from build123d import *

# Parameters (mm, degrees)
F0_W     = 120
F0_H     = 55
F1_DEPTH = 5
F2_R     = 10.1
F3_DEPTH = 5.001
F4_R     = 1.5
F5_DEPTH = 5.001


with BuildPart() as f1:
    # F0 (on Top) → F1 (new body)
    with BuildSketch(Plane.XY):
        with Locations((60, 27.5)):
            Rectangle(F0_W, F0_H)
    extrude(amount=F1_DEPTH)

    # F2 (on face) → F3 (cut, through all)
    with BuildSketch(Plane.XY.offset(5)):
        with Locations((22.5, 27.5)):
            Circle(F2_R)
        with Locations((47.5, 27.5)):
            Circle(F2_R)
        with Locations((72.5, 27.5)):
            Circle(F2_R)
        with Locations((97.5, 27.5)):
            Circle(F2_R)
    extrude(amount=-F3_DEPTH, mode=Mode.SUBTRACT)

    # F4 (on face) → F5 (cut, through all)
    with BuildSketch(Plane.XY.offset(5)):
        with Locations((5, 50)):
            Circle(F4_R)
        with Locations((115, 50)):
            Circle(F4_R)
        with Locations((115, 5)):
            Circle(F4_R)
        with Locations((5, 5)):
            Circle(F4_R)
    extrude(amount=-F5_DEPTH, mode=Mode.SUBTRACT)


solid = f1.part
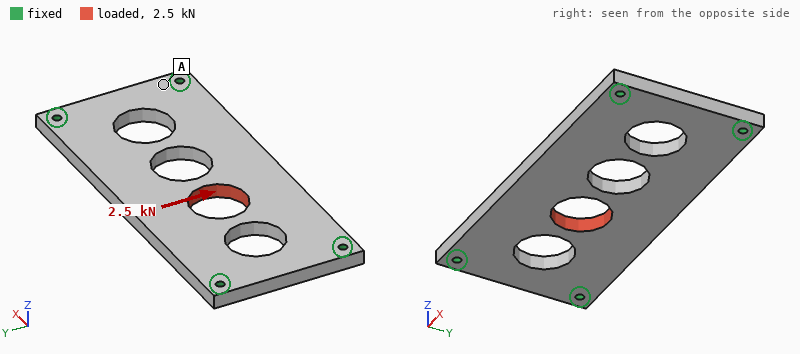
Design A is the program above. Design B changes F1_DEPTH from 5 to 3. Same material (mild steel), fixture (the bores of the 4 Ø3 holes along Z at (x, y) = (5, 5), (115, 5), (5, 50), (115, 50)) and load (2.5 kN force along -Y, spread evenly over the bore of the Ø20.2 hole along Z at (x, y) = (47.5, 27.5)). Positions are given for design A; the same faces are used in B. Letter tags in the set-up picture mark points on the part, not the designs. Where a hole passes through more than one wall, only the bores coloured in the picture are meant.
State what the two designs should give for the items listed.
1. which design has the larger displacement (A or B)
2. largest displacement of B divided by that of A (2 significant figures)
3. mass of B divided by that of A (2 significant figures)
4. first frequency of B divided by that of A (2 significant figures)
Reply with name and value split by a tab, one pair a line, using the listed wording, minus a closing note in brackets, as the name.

which design has the larger displacement	B
largest displacement of B divided by that of A	1.7
mass of B divided by that of A	0.60
first frequency of B divided by that of A	0.62
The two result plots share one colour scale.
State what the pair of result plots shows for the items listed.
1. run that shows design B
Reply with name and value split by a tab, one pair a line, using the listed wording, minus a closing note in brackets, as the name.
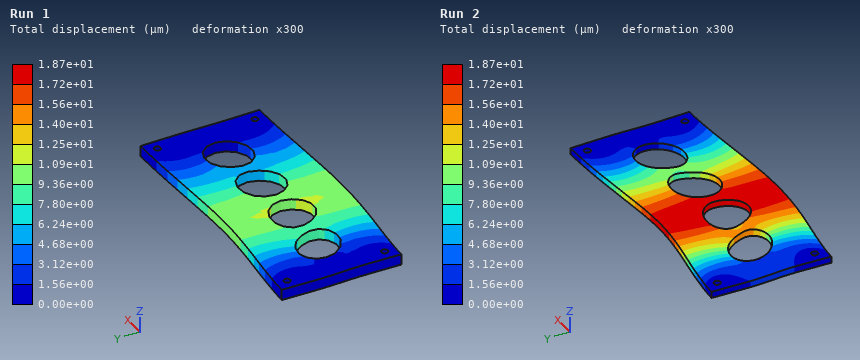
run that shows design B	Run 2
